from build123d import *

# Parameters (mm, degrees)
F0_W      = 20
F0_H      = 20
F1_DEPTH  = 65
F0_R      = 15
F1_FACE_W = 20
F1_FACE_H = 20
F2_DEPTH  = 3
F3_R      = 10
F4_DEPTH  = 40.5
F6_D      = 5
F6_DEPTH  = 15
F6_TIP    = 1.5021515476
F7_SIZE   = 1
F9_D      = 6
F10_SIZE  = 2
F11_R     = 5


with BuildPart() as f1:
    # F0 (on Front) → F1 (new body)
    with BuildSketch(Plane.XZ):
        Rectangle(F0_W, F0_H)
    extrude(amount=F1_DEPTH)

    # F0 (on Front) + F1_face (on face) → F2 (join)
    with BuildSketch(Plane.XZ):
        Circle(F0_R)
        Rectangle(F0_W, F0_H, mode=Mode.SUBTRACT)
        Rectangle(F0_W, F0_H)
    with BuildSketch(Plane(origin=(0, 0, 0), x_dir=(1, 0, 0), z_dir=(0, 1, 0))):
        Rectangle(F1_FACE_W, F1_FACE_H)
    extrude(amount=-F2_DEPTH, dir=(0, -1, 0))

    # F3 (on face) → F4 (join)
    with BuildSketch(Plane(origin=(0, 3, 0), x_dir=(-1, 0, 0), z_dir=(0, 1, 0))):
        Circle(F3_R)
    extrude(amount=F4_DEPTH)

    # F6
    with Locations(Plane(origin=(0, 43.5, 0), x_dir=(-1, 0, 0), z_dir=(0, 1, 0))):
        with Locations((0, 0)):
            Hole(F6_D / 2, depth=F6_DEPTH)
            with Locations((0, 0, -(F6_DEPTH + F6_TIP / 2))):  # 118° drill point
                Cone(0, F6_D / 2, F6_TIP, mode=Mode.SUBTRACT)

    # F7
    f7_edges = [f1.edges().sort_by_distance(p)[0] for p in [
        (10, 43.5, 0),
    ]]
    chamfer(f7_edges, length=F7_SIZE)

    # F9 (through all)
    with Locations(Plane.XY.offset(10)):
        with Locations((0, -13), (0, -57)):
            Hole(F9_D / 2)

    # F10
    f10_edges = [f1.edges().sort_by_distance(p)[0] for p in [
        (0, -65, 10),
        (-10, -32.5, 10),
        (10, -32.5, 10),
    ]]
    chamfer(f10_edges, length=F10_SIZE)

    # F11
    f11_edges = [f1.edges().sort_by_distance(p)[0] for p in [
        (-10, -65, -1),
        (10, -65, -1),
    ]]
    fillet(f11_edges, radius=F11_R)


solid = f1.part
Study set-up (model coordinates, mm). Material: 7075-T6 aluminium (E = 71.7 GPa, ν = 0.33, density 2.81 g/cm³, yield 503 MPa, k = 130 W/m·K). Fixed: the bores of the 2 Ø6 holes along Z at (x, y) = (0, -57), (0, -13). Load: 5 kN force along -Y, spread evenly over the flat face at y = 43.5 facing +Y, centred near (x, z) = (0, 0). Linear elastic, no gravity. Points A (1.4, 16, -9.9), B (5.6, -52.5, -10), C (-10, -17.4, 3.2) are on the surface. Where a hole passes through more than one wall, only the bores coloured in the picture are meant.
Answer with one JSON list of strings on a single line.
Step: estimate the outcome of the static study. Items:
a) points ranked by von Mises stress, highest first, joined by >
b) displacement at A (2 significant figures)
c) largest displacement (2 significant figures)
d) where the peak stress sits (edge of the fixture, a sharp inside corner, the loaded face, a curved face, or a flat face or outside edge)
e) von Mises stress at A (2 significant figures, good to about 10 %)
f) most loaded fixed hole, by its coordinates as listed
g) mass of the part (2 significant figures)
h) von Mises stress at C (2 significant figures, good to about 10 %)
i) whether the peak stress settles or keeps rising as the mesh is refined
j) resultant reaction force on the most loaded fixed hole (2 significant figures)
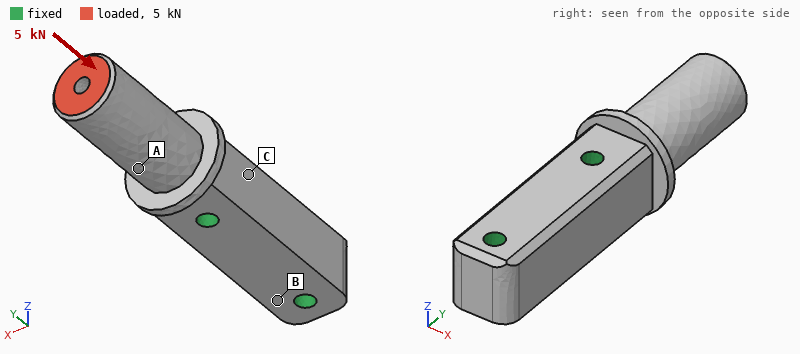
["A > C > B", "6.0 µm", "13 µm", "edge of the fixture", "16 MPa", "(0, -13)", "110 g", "5.2 MPa", "keeps rising", "4.7 kN"]
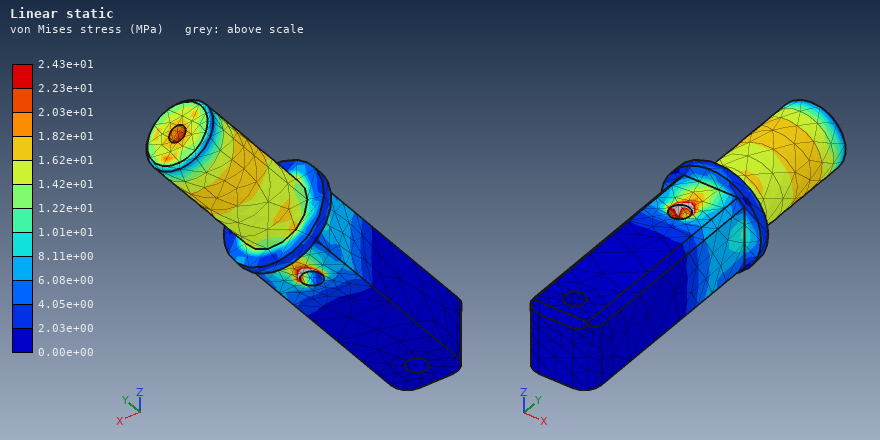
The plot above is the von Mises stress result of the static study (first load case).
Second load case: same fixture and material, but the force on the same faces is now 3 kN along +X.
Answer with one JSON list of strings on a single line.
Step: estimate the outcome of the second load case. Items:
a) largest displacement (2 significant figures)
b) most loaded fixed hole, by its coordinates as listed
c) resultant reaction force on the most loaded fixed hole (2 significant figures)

["0.34 mm", "(0, -13)", "5.0 kN"]
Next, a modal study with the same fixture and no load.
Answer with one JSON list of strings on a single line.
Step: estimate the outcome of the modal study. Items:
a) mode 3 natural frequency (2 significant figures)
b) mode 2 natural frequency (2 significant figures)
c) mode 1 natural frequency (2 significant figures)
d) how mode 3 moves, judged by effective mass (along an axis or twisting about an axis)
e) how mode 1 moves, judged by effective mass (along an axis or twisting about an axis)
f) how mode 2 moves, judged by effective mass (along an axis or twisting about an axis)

["15 kHz", "4900 Hz", "4300 Hz", "twisting about Y", "along X", "along Z"]
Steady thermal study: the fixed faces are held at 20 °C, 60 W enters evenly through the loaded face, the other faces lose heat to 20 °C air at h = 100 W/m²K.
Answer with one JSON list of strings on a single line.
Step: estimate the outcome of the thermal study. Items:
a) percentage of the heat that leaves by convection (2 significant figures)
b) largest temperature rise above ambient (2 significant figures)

["23 %", "69 K"]
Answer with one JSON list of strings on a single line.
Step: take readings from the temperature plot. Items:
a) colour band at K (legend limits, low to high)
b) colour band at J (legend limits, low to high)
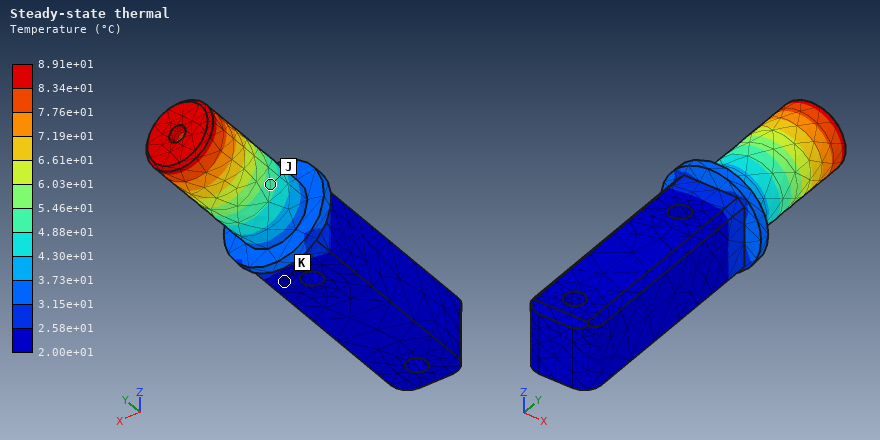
["2.00e+01 to 2.58e+01 °C", "4.88e+01 to 5.46e+01 °C"]
